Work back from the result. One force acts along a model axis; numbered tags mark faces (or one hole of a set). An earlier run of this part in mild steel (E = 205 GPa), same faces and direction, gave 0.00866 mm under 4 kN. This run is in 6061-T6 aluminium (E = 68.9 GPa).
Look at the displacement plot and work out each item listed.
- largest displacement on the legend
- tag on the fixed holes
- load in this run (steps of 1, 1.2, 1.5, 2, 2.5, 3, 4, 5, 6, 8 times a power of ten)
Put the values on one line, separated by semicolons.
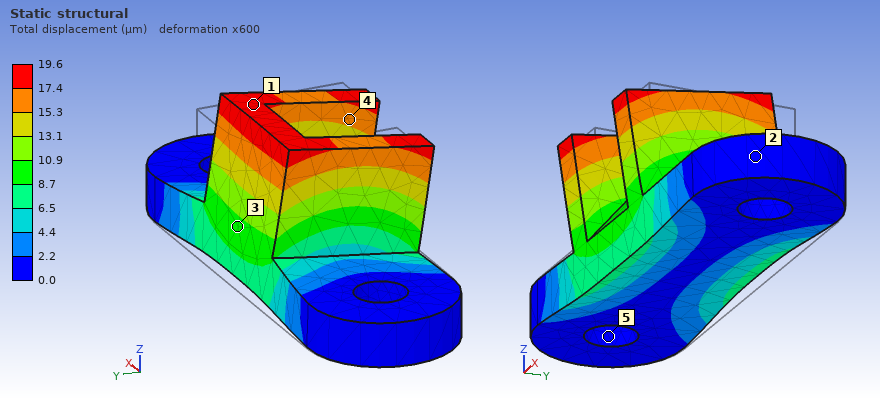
19.6 µm; 5; 3 kN
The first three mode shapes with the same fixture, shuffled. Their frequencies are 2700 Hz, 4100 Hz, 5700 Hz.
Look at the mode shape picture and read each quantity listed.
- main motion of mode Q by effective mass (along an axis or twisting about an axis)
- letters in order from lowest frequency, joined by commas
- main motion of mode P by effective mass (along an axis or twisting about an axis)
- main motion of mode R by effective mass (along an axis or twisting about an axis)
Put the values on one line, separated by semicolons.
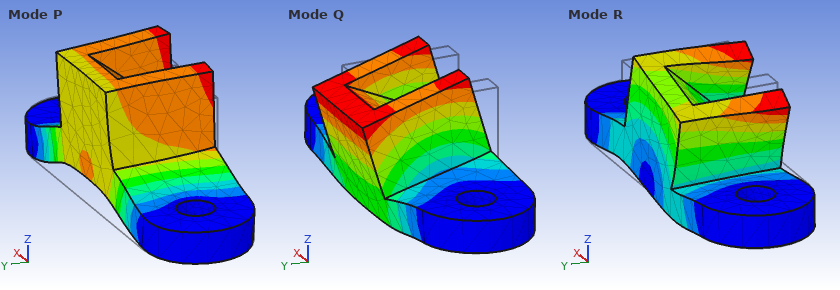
along Y; Q, P, R; along Z; along X
